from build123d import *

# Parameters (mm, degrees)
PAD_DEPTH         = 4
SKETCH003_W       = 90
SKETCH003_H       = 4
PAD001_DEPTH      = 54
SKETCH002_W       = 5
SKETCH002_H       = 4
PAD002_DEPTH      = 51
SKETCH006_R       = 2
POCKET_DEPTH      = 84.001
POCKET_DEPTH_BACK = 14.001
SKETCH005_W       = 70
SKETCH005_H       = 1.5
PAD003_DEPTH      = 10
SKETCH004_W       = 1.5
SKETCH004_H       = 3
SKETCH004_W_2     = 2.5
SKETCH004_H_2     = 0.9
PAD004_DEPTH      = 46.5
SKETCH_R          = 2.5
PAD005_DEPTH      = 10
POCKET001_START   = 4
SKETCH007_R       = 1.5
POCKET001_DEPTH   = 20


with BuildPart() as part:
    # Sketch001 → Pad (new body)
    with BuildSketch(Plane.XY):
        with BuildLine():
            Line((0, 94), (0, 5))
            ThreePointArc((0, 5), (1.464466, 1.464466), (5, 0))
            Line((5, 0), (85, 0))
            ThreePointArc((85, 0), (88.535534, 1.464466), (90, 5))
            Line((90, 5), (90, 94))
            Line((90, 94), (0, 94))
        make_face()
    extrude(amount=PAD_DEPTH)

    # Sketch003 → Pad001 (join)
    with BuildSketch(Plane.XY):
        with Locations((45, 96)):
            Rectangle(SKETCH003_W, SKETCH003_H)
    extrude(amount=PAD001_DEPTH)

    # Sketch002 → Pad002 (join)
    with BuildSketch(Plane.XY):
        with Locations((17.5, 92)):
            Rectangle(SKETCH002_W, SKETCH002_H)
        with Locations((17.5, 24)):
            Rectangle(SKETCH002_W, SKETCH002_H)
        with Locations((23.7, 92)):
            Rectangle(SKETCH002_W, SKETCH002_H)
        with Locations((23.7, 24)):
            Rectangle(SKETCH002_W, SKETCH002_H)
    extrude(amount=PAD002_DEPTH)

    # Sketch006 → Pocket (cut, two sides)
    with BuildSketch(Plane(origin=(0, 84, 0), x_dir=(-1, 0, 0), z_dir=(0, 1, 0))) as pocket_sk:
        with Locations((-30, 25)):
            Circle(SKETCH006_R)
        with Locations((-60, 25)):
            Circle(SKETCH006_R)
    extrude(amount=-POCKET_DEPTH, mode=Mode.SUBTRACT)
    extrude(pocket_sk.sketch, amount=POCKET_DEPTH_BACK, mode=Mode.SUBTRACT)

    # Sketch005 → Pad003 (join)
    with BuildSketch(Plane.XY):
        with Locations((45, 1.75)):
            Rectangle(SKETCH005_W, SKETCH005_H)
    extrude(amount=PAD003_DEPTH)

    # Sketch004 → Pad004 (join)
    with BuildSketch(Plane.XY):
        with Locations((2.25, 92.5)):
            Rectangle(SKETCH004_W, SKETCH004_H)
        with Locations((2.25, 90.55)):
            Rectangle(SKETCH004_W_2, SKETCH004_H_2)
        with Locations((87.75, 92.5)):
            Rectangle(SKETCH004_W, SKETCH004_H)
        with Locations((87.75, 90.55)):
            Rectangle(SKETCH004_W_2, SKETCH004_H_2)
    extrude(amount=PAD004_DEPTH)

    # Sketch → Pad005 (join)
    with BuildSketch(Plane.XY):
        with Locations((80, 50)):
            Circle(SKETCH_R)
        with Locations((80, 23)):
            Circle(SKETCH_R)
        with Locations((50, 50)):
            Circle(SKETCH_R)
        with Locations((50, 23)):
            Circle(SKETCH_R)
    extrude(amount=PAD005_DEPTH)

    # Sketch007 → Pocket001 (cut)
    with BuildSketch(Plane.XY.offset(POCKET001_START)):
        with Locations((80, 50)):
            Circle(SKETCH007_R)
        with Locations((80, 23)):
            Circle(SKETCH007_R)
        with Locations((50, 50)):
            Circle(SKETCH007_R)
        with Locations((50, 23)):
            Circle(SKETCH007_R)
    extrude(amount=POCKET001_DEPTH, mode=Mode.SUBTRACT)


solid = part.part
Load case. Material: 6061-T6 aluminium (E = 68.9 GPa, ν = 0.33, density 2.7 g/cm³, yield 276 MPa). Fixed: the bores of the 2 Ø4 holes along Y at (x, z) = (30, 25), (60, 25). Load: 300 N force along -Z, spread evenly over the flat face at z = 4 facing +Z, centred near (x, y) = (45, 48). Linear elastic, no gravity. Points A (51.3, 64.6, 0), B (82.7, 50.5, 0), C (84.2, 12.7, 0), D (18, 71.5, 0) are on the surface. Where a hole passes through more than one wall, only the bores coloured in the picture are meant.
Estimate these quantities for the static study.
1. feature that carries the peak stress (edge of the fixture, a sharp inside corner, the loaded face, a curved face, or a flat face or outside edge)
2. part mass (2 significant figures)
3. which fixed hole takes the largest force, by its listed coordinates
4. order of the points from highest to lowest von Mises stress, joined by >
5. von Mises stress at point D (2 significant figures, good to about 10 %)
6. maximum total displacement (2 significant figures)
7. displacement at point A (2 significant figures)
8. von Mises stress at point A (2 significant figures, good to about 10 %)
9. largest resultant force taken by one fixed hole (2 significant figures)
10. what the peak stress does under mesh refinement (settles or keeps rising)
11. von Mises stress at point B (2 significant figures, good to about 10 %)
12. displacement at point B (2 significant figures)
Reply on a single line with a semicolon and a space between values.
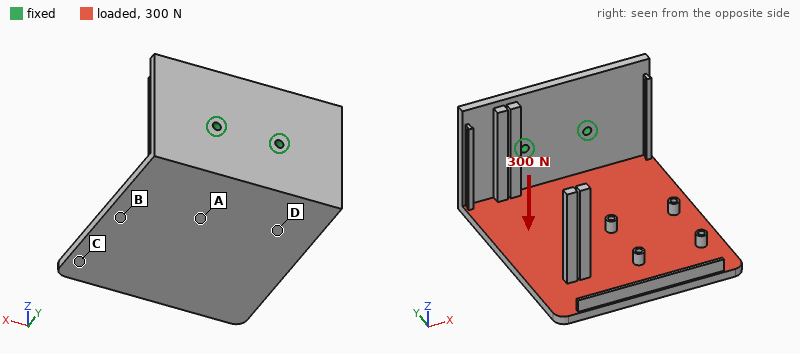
edge of the fixture; 160 g; (60, 25); D > A > B > C; 33 MPa; 1.6 mm; 0.39 mm; 24 MPa; 170 N; keeps rising; 15 MPa; 0.62 mm
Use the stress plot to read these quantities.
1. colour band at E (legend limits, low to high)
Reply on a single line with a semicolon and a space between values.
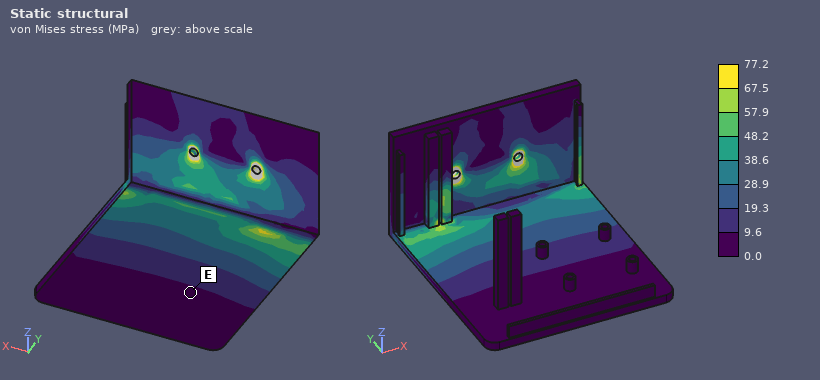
0.0 to 9.6 MPa
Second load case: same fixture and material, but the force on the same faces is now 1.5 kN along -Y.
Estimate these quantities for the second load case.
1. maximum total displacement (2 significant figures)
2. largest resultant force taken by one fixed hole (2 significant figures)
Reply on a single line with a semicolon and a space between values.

0.75 mm; 770 N
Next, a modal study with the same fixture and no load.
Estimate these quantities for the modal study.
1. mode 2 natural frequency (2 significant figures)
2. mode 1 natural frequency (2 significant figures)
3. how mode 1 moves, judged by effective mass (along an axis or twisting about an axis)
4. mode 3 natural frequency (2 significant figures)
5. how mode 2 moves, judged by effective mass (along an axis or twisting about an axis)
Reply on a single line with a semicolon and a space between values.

560 Hz; 260 Hz; along Z; 870 Hz; along X
